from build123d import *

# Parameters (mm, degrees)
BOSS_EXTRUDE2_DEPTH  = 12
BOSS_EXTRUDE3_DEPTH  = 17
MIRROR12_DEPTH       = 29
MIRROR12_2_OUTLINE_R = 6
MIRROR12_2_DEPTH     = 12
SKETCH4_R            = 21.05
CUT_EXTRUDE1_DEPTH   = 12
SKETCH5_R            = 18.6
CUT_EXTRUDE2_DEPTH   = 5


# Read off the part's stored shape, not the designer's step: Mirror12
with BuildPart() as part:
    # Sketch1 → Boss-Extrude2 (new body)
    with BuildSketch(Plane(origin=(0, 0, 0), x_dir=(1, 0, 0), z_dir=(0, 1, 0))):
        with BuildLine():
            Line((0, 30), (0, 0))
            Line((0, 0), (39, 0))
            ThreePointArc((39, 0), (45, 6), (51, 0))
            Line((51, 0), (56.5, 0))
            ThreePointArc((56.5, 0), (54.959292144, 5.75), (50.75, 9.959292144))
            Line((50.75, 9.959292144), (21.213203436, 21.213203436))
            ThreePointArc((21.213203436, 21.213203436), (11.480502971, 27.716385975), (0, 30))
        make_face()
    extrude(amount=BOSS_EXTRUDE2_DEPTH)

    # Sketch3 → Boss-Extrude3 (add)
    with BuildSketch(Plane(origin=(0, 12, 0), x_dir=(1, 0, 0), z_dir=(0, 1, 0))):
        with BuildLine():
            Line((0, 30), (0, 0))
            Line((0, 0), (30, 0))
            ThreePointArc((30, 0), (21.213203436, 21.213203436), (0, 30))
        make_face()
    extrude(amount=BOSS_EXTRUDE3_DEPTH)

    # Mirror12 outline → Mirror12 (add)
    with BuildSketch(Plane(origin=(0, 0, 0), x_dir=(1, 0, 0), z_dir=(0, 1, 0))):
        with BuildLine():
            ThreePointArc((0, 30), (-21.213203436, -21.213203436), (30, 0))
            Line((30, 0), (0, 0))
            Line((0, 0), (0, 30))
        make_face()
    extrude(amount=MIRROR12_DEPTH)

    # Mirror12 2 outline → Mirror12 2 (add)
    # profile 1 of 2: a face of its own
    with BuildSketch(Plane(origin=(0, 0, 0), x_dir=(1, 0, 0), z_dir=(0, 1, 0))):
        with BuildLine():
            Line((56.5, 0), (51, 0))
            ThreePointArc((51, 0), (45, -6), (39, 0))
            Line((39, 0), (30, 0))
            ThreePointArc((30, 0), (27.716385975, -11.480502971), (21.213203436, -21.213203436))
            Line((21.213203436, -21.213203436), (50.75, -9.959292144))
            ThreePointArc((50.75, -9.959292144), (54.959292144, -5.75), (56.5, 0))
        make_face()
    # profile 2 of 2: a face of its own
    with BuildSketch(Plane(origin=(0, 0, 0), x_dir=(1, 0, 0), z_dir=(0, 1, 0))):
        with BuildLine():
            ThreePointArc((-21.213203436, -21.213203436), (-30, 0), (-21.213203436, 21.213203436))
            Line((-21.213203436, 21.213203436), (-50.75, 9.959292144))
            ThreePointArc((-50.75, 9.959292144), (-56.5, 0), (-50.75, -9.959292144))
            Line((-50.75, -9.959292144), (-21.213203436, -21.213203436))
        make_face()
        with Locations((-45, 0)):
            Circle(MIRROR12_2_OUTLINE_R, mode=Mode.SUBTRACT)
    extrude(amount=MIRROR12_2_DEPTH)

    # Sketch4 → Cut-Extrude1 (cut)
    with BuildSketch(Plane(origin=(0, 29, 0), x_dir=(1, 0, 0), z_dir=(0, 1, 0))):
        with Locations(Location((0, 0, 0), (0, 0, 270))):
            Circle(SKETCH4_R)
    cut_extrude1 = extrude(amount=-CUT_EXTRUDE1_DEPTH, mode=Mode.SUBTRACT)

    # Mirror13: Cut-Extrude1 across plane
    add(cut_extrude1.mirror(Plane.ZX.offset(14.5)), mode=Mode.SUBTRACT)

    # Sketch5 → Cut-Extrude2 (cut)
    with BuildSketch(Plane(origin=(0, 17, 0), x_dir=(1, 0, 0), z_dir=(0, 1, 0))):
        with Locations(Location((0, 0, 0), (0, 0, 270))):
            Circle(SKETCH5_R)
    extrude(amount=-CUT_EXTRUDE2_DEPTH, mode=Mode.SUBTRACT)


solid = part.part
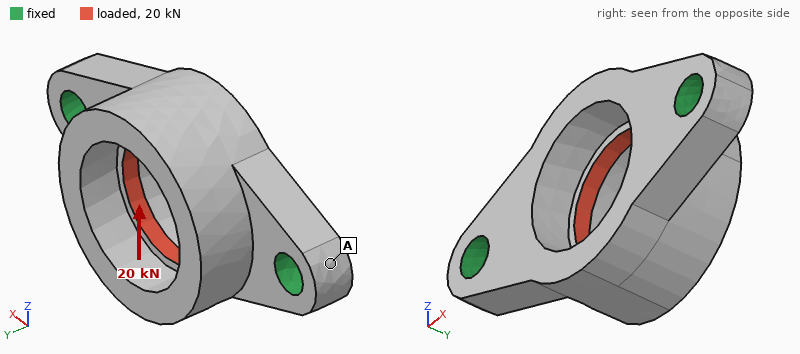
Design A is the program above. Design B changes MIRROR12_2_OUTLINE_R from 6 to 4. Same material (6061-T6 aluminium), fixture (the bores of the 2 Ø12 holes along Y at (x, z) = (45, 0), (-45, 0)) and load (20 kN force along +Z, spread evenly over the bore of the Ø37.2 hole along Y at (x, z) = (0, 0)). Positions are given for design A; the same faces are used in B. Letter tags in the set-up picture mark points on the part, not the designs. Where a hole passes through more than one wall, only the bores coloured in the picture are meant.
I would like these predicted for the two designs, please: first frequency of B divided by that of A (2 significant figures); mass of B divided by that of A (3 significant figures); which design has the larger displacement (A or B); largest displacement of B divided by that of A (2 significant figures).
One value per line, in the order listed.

0.94
1.01
B
1.1
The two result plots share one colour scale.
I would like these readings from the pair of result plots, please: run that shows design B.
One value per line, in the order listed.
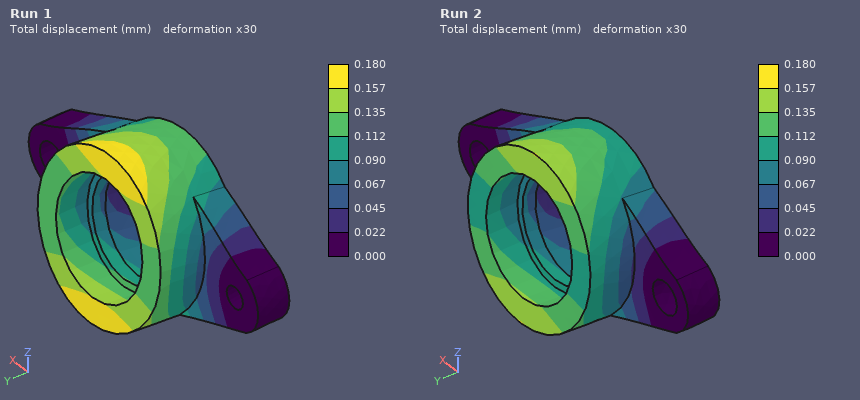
Run 1
